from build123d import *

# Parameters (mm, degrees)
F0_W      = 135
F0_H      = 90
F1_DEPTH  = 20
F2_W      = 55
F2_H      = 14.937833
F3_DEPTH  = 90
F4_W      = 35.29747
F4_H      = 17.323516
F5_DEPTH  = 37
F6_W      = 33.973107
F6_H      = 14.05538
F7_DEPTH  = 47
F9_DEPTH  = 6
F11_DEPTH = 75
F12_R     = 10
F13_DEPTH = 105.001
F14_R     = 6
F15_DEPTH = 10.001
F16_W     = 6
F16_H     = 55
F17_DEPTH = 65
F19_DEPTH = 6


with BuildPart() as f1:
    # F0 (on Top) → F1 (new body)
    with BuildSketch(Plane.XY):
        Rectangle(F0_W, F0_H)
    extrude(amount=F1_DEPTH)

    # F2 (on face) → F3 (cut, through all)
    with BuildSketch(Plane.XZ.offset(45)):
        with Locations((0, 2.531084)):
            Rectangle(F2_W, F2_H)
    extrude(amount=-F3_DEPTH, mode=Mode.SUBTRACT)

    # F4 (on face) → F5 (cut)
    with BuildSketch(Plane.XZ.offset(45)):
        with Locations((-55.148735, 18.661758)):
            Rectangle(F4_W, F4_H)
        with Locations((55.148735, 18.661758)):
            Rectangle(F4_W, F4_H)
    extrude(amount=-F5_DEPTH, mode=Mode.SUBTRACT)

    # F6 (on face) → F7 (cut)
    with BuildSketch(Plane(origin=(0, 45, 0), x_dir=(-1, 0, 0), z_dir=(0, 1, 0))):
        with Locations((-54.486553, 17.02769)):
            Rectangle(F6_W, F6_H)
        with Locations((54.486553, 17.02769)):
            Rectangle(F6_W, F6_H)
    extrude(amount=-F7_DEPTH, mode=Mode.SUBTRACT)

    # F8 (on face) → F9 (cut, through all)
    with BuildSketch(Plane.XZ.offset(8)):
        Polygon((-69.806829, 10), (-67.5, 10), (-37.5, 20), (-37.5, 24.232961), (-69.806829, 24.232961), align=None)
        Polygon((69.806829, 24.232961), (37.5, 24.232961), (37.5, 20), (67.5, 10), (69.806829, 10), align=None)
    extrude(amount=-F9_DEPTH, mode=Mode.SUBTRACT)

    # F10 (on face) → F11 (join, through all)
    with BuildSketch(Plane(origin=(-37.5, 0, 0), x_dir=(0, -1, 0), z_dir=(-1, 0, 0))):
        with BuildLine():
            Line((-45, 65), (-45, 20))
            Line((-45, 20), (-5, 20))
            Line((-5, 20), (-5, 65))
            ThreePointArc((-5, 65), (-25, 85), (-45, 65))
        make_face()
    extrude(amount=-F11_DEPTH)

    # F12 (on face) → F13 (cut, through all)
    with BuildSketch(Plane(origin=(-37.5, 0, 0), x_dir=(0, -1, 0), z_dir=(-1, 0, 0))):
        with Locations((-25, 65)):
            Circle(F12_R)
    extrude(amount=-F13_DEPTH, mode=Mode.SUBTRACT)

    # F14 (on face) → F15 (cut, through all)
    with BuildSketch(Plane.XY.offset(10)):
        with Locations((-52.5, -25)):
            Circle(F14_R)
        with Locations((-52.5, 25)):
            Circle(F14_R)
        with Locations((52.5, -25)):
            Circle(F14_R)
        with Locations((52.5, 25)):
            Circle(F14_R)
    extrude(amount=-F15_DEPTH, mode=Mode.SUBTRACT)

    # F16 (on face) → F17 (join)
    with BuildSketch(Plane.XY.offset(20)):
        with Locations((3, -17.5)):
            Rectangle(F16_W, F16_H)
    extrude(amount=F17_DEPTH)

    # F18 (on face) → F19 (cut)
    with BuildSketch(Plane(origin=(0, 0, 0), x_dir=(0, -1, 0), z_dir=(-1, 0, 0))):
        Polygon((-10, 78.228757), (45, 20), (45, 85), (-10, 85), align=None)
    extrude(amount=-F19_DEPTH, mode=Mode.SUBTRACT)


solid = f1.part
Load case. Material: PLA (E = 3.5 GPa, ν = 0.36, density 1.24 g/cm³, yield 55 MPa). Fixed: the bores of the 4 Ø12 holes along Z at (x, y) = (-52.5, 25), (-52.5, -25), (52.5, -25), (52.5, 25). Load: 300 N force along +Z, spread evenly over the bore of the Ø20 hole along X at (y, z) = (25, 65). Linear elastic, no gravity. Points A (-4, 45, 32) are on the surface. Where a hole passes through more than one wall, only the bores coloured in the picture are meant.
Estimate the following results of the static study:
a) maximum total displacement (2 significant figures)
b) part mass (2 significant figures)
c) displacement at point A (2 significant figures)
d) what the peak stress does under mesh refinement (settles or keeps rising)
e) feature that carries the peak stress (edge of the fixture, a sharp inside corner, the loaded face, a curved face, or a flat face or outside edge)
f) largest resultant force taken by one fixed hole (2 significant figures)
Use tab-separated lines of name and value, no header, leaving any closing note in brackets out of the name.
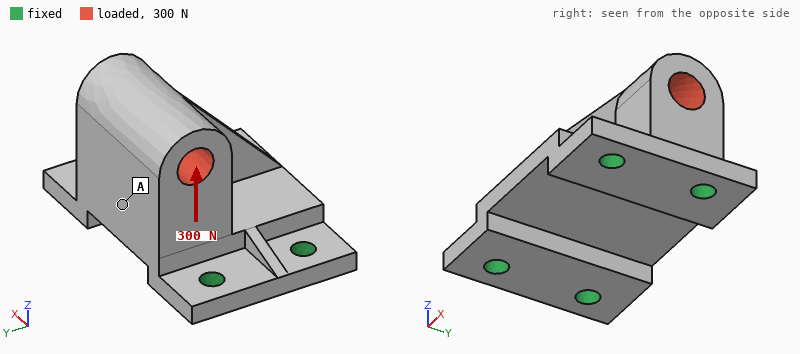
maximum total displacement	25 µm
part mass	380 g
displacement at point A	20 µm
what the peak stress does under mesh refinement	keeps rising
feature that carries the peak stress	edge of the fixture
largest resultant force taken by one fixed hole	170 N
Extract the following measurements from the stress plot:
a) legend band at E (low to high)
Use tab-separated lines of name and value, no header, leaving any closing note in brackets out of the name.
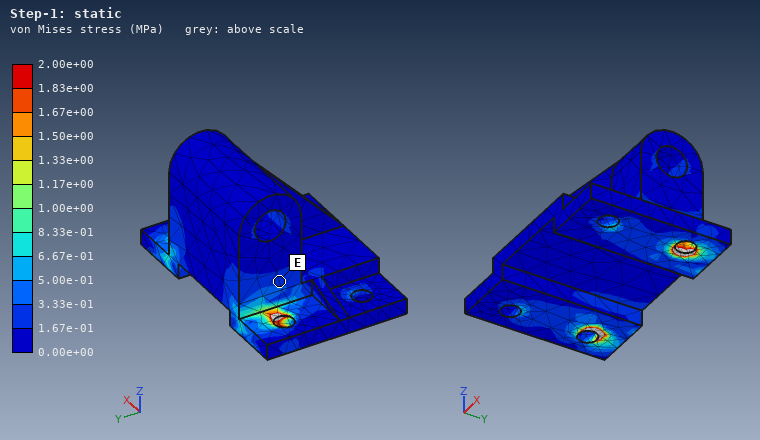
legend band at E	1.67e-01 to 3.33e-01 MPa
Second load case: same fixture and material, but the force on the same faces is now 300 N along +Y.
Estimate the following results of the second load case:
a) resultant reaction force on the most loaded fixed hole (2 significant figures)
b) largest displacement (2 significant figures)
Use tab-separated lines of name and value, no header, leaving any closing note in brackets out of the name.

resultant reaction force on the most loaded fixed hole	290 N
largest displacement	0.11 mm
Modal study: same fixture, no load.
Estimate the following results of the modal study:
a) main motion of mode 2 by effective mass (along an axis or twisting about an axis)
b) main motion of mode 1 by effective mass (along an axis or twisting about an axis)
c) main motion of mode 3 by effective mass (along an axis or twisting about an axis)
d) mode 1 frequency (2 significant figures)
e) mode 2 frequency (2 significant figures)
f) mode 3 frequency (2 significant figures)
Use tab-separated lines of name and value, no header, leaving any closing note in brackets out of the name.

main motion of mode 2 by effective mass	along X
main motion of mode 1 by effective mass	along Y
main motion of mode 3 by effective mass	along Z
mode 1 frequency	810 Hz
mode 2 frequency	1400 Hz
mode 3 frequency	1600 Hz
